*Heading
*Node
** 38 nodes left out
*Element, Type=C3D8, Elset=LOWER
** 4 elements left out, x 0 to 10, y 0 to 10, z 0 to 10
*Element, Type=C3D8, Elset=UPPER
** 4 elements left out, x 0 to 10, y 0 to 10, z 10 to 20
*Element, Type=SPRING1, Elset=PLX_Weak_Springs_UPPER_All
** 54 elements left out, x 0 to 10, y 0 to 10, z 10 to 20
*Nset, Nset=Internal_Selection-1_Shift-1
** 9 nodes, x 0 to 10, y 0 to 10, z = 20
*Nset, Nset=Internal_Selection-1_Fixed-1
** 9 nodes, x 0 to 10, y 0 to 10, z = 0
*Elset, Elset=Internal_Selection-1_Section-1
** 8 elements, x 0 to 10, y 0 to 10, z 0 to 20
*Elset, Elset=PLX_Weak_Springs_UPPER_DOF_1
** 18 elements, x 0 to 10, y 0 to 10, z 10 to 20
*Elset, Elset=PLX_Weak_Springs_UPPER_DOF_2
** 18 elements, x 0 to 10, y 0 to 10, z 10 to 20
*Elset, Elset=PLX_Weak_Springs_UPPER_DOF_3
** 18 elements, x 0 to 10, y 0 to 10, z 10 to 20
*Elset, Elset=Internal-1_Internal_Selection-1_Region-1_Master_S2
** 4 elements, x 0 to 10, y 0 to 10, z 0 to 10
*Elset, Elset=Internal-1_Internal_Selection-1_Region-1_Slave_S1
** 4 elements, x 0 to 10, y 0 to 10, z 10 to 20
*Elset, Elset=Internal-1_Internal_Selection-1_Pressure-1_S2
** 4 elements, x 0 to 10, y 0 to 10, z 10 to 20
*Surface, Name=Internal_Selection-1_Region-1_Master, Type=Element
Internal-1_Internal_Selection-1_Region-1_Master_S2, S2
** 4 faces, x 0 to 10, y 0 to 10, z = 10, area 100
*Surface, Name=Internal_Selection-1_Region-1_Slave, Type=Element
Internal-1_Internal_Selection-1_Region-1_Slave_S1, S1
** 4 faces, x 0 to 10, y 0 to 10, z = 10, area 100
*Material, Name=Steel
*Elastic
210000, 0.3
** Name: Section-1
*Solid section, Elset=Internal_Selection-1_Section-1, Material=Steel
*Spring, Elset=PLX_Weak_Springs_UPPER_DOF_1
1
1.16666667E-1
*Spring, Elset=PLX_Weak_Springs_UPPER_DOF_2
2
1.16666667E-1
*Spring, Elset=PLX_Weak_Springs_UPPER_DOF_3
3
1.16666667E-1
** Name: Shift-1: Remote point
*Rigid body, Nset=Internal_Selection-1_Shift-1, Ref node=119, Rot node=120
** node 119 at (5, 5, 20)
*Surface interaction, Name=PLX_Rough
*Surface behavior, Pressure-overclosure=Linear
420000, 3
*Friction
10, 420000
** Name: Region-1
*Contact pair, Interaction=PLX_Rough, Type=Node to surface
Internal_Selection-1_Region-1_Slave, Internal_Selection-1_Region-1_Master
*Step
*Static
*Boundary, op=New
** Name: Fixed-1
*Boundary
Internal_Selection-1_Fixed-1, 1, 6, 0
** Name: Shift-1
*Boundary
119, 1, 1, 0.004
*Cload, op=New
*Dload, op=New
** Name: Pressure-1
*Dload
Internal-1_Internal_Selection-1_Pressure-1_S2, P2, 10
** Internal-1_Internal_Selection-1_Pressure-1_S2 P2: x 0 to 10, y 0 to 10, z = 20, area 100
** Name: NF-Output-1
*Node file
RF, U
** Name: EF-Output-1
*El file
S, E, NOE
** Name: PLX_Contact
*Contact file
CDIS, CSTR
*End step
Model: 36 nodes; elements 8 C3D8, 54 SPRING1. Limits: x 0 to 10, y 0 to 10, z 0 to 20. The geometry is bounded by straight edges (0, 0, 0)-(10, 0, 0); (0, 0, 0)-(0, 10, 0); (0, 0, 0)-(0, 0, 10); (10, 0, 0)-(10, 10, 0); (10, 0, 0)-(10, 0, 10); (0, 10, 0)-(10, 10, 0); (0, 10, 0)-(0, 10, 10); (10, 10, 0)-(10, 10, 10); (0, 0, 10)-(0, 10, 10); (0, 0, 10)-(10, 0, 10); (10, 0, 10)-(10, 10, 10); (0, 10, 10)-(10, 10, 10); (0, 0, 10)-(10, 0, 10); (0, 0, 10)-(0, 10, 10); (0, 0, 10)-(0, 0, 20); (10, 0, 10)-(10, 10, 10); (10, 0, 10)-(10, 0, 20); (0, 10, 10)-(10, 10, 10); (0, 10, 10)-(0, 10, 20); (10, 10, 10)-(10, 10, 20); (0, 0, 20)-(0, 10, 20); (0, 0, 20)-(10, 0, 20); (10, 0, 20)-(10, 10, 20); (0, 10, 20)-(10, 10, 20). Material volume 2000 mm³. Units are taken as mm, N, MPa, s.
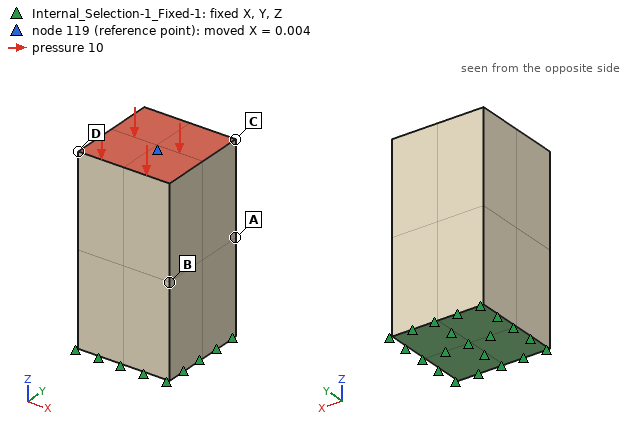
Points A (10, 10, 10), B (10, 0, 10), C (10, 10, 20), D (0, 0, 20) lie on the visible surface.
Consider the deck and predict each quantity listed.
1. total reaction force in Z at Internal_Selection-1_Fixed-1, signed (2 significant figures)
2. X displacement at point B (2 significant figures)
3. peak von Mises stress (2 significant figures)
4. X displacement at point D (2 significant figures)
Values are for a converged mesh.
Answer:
1000 N
0.0014 mm
30 MPa
0.0040 mm
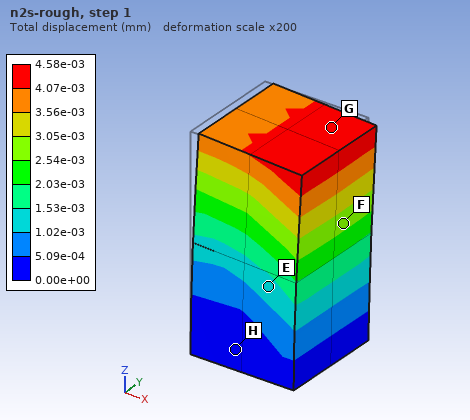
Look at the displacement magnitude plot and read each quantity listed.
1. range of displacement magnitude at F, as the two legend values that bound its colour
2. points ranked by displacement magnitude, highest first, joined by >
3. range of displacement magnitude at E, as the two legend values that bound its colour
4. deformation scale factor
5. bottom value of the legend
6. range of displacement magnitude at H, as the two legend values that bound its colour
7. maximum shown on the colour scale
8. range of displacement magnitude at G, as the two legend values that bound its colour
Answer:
2.54e-03 to 3.05e-03 mm
G > F > E > H
1.02e-03 to 1.53e-03 mm
200
0.00e+00 mm
0.00e+00 to 5.09e-04 mm
4.58e-03 mm
4.07e-03 to 4.58e-03 mm
